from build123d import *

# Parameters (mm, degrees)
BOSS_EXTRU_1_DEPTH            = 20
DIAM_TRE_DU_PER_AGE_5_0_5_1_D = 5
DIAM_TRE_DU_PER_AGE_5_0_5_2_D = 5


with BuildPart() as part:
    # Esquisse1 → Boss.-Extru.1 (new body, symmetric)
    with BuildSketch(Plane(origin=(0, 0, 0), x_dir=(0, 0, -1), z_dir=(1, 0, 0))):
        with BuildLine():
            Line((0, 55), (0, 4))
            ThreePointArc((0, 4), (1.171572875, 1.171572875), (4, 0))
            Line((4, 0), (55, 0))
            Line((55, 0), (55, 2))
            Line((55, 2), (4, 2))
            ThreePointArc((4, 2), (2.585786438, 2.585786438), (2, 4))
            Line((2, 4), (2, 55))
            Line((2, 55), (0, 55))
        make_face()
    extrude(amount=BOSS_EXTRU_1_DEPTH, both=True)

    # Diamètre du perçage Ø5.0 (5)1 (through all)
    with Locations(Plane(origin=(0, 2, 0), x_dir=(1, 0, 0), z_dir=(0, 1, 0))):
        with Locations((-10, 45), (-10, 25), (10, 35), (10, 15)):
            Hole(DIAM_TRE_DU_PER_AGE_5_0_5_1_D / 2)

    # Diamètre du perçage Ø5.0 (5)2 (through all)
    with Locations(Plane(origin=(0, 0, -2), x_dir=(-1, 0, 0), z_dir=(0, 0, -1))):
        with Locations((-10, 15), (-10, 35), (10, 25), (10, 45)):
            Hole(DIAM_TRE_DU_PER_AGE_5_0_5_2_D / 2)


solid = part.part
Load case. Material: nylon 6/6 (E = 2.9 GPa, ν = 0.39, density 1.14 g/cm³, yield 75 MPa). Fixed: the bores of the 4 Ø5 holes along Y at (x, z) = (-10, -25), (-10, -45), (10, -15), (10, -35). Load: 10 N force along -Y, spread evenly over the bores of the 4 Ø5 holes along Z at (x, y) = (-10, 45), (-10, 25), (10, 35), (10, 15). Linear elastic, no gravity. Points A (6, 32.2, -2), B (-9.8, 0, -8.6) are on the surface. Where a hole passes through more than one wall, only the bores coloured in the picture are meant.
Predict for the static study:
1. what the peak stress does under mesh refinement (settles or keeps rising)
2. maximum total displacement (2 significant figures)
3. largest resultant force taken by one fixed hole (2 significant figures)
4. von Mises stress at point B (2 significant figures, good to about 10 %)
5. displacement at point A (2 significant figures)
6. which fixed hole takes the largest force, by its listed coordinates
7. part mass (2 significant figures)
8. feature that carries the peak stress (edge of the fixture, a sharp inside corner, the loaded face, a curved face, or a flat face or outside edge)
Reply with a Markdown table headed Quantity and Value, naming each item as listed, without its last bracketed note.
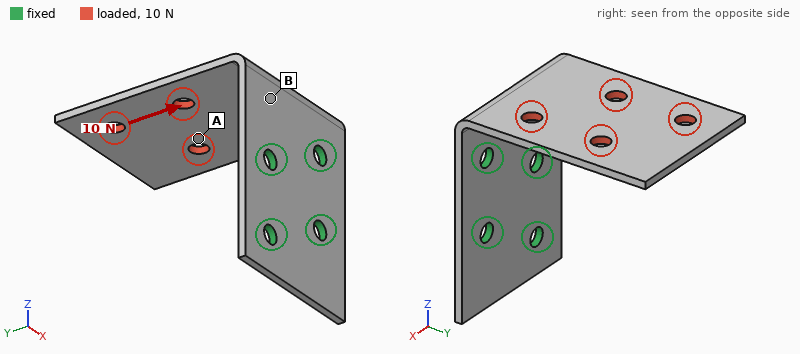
| Quantity | Value |
|---|---|
| what the peak stress does under mesh refinement | keeps rising |
| maximum total displacement | 0.92 mm |
| largest resultant force taken by one fixed hole | 8.7 N |
| von Mises stress at point B | 1.7 MPa |
| displacement at point A | 0.50 mm |
| which fixed hole takes the largest force, by its listed coordinates | (10, -15) |
| part mass | 9.4 g |
| feature that carries the peak stress | edge of the fixture |
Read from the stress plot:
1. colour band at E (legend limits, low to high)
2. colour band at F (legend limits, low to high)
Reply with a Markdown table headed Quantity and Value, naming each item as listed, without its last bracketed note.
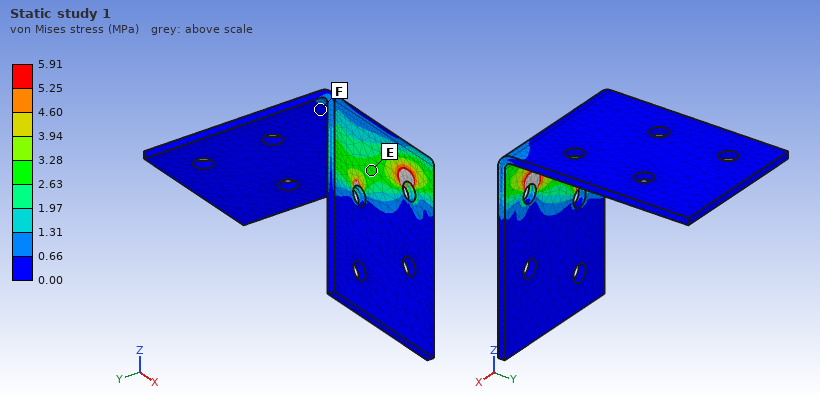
| Quantity | Value |
|---|---|
| colour band at E | 2.63 to 3.28 MPa |
| colour band at F | 0.00 to 0.66 MPa |
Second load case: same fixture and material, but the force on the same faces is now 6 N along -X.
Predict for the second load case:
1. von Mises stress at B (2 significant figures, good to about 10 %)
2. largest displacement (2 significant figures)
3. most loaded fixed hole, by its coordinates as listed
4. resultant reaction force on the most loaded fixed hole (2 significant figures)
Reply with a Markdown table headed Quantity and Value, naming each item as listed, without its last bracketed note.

| Quantity | Value |
|---|---|
| von Mises stress at B | 2.0 MPa |
| largest displacement | 0.82 mm |
| most loaded fixed hole, by its coordinates as listed | (10, -15) |
| resultant reaction force on the most loaded fixed hole | 7.5 N |
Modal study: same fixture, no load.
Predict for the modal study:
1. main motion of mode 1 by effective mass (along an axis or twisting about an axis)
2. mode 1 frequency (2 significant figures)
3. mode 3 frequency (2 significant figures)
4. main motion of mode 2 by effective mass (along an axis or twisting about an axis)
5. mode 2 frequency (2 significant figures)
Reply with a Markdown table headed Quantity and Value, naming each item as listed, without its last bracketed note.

| Quantity | Value |
|---|---|
| main motion of mode 1 by effective mass | along Z |
| mode 1 frequency | 130 Hz |
| mode 3 frequency | 510 Hz |
| main motion of mode 2 by effective mass | along X |
| mode 2 frequency | 260 Hz |
